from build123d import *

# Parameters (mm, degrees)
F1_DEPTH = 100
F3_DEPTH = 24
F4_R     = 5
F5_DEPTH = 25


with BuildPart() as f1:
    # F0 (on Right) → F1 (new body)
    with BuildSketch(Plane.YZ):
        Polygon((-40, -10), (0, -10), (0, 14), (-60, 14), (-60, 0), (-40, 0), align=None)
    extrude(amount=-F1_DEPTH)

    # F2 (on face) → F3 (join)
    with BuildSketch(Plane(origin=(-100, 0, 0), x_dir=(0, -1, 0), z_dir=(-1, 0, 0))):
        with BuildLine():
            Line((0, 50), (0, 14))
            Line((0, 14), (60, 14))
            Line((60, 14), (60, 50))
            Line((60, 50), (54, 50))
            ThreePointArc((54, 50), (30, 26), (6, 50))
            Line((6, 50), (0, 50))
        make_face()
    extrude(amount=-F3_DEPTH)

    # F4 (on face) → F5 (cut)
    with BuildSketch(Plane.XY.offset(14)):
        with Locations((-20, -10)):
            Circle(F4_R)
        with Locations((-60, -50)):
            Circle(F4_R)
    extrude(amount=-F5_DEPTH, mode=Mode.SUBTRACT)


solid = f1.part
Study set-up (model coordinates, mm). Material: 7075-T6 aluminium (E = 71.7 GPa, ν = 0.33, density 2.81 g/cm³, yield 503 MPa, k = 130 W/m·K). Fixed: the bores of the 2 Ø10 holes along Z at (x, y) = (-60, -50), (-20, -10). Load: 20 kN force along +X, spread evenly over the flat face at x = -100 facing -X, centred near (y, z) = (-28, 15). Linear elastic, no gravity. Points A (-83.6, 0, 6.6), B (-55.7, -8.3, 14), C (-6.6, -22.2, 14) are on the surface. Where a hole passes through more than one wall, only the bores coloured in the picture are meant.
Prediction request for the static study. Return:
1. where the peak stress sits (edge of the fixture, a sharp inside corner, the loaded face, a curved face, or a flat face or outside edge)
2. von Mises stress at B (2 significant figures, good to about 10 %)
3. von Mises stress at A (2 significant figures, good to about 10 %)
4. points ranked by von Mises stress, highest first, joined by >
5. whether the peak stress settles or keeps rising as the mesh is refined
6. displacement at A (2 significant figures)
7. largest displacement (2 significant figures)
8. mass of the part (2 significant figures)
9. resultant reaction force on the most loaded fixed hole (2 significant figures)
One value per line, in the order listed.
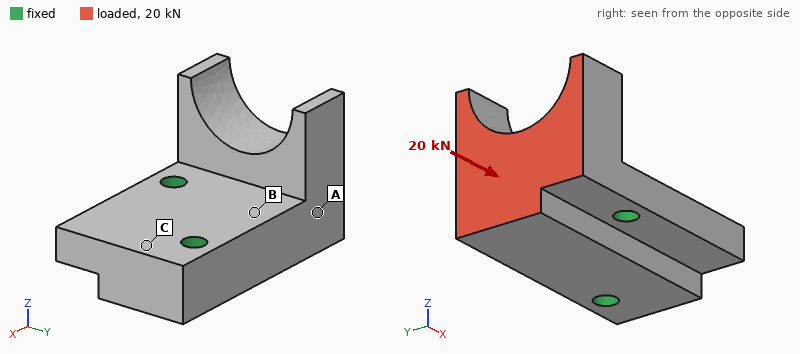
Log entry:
edge of the fixture
51 MPa
27 MPa
B > A > C
keeps rising
0.068 mm
0.19 mm
420 g
11 kN
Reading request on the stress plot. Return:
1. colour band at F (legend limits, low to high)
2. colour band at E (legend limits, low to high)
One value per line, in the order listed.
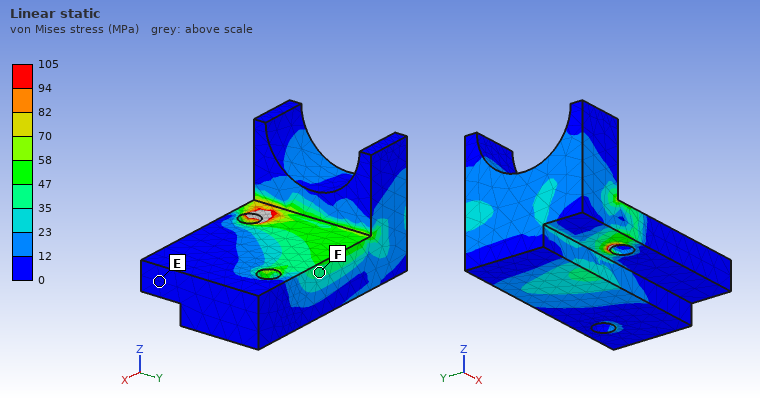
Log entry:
35 to 47 MPa
0 to 12 MPa
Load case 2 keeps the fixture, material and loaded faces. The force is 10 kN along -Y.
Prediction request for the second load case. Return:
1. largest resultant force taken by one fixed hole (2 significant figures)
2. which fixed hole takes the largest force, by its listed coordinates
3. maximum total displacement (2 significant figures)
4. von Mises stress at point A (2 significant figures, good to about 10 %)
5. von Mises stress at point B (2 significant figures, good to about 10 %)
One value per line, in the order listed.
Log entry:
14 kN
(-60, -50)
78 µm
12 MPa
22 MPa
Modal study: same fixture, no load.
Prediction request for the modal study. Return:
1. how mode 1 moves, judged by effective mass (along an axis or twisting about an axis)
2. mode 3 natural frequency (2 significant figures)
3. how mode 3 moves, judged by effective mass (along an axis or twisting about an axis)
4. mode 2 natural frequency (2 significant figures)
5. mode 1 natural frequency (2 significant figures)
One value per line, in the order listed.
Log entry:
along Z
8100 Hz
along Y
5500 Hz
3100 Hz
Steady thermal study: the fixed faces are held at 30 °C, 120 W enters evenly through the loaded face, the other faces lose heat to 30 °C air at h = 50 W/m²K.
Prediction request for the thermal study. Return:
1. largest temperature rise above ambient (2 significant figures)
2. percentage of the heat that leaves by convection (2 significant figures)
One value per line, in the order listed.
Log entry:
36 K
12 %
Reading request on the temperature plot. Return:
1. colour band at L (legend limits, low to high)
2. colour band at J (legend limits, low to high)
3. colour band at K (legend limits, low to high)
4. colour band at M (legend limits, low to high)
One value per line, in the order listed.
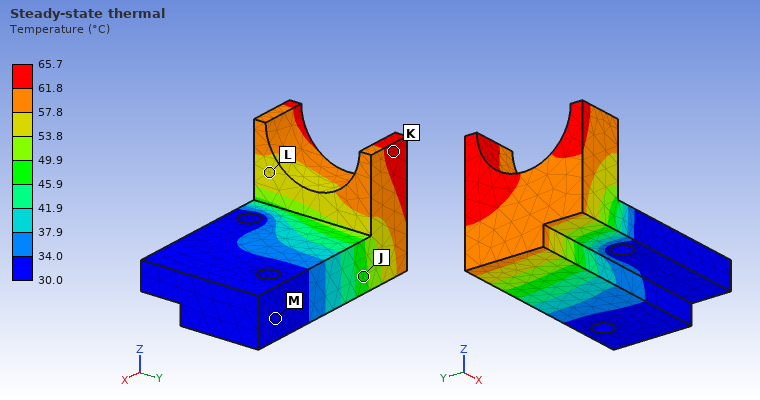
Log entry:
53.8 to 57.8 °C
45.9 to 49.9 °C
61.8 to 65.7 °C
30.0 to 34.0 °C
